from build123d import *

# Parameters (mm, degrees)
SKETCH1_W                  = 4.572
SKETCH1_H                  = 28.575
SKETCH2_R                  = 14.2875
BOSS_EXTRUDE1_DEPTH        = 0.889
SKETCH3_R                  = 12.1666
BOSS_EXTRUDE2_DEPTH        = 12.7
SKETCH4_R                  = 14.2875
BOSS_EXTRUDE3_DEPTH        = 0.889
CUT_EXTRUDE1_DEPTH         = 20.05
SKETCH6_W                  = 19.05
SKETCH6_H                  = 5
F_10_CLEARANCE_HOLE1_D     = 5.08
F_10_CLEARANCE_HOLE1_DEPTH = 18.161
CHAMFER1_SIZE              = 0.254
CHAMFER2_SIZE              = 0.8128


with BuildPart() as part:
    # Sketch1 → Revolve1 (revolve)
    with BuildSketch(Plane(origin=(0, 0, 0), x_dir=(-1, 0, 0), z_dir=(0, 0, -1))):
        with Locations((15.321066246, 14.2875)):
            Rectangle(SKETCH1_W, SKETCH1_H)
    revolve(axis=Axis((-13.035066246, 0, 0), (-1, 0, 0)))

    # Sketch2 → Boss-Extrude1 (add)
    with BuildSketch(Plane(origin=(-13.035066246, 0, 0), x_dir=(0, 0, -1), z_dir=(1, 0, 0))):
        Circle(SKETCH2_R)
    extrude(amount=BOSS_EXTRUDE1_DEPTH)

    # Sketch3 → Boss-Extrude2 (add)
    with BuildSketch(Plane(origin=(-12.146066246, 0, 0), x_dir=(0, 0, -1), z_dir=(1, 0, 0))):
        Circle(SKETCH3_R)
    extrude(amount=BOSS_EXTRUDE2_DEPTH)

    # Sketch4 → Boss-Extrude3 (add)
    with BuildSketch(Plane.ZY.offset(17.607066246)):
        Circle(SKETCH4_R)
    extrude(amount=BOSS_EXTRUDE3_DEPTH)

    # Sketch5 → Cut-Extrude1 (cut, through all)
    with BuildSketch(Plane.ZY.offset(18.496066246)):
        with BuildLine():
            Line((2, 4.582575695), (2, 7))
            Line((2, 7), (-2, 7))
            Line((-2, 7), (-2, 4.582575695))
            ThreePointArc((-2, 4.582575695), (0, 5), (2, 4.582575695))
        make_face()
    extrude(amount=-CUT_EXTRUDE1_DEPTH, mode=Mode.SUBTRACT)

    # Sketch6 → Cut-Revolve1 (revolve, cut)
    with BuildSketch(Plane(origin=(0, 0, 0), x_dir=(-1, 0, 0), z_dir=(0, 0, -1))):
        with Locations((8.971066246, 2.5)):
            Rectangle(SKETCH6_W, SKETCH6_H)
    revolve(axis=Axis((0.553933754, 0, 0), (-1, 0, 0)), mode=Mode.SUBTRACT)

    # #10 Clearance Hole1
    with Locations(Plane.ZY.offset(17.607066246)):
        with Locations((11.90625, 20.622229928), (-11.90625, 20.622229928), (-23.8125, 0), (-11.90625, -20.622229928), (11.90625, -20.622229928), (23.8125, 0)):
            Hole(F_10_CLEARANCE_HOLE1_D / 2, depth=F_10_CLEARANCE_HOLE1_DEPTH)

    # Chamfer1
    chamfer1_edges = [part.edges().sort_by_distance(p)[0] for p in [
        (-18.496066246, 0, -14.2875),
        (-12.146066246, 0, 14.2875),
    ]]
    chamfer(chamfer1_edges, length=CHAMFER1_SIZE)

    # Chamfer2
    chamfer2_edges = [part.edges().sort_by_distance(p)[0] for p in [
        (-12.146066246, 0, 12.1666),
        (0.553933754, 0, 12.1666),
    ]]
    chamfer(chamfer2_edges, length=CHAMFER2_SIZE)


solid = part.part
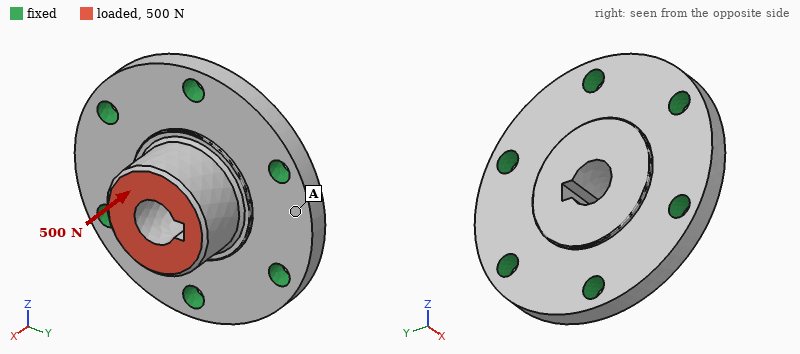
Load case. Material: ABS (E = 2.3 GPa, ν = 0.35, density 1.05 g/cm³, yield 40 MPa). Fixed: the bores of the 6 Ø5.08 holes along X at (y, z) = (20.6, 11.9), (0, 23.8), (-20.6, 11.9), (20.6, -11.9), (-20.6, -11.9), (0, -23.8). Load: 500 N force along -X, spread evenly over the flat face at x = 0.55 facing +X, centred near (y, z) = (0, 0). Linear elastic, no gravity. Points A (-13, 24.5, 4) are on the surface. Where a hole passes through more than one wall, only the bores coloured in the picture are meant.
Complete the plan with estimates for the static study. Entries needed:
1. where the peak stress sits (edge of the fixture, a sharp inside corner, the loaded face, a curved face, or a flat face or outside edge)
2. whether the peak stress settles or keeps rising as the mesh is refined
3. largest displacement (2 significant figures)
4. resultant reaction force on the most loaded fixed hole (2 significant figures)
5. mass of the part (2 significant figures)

edge of the fixture
keeps rising
64 µm
91 N
17 g
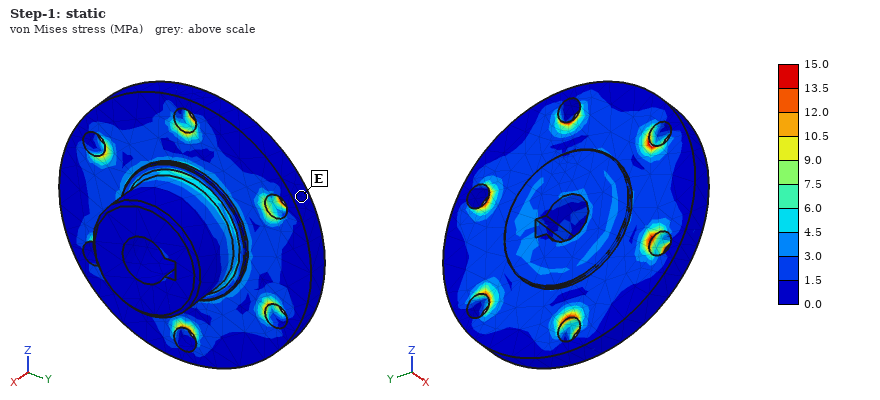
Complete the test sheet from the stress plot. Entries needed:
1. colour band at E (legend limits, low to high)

0.0 to 1.5 MPa
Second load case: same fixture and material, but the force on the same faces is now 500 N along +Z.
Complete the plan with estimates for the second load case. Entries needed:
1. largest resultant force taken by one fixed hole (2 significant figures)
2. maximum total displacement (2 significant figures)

190 N
0.14 mm
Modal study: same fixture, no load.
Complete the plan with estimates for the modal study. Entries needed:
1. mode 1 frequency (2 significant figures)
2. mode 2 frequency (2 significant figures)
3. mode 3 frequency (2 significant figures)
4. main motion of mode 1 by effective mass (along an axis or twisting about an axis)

4900 Hz
5900 Hz
6000 Hz
along X
